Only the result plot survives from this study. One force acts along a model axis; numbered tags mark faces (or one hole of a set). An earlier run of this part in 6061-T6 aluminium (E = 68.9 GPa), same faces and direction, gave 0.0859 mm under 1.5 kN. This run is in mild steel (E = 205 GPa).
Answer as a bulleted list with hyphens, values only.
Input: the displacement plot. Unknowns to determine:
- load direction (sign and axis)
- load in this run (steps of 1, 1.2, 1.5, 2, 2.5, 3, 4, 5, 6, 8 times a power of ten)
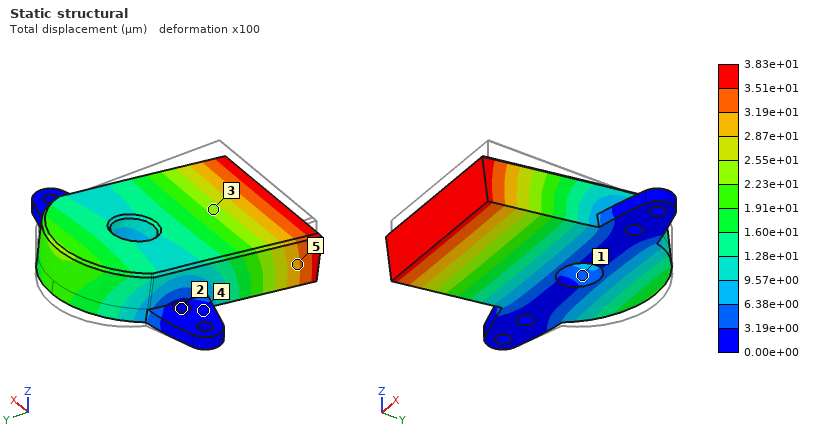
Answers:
- -Y
- 2 kN
